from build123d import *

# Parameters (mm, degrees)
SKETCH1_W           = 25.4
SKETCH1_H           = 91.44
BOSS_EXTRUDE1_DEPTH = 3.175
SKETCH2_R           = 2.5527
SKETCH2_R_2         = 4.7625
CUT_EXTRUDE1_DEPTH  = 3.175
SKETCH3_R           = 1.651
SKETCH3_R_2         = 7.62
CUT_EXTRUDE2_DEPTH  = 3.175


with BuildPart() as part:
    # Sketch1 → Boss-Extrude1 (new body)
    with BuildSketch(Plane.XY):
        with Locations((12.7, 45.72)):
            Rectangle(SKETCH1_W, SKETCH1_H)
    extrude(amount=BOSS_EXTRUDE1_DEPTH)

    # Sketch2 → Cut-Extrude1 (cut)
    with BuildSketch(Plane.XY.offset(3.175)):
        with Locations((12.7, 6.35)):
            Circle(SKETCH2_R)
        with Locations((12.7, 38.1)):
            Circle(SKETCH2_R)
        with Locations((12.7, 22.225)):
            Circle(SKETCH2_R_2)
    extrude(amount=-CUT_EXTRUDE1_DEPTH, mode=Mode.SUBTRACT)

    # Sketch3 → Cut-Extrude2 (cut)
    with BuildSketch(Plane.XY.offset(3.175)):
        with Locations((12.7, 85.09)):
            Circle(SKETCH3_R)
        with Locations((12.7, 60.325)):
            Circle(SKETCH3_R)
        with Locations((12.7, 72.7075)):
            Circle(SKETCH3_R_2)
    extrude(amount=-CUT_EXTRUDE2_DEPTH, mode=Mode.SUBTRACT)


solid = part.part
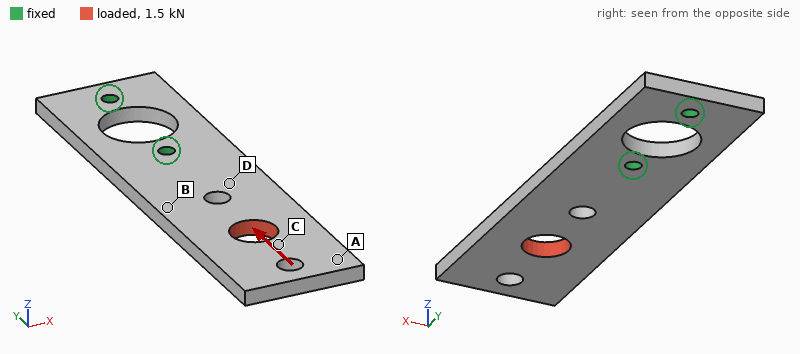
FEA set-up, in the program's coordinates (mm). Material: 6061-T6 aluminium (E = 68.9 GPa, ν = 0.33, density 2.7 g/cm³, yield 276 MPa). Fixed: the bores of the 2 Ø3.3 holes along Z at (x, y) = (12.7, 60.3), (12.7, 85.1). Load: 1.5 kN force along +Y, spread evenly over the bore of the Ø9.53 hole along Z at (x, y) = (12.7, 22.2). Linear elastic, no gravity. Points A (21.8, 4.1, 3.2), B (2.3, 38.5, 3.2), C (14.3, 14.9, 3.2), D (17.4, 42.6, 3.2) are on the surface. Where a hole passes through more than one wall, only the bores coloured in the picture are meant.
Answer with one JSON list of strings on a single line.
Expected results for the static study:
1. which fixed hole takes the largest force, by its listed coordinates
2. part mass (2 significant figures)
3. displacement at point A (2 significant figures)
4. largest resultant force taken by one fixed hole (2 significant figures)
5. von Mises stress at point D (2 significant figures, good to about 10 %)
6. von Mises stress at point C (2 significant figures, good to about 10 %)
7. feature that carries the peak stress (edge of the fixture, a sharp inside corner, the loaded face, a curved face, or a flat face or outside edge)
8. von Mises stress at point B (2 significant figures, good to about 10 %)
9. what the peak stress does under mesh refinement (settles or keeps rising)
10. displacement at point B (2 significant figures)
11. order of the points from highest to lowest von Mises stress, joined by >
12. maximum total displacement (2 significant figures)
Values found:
["(12.7, 60.3)", "17 g", "14 µm", "1.3 kN", "25 MPa", "13 MPa", "edge of the fixture", "19 MPa", "keeps rising", "8.8 µm", "D > B > C > A", "17 µm"]
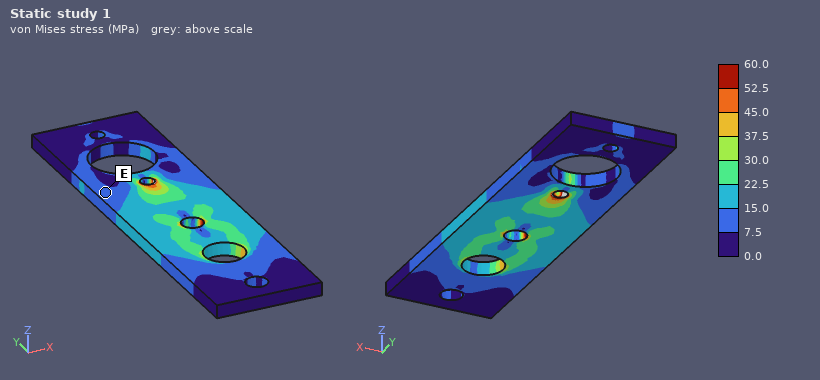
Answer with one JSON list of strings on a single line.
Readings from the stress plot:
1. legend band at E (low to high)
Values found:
["7.5 to 15.0 MPa"]
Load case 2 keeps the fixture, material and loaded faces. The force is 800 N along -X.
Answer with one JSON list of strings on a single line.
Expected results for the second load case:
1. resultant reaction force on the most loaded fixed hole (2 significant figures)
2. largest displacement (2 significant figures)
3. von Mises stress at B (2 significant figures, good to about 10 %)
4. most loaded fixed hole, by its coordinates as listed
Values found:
["1.5 kN", "0.29 mm", "35 MPa", "(12.7, 60.3)"]
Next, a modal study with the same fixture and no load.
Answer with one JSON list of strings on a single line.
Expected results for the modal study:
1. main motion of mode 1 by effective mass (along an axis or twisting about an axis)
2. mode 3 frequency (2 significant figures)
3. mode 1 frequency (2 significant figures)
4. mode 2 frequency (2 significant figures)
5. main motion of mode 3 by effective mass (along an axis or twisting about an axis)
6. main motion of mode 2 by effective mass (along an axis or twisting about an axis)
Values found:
["along Z", "3300 Hz", "710 Hz", "2900 Hz", "along X", "twisting about Y"]
